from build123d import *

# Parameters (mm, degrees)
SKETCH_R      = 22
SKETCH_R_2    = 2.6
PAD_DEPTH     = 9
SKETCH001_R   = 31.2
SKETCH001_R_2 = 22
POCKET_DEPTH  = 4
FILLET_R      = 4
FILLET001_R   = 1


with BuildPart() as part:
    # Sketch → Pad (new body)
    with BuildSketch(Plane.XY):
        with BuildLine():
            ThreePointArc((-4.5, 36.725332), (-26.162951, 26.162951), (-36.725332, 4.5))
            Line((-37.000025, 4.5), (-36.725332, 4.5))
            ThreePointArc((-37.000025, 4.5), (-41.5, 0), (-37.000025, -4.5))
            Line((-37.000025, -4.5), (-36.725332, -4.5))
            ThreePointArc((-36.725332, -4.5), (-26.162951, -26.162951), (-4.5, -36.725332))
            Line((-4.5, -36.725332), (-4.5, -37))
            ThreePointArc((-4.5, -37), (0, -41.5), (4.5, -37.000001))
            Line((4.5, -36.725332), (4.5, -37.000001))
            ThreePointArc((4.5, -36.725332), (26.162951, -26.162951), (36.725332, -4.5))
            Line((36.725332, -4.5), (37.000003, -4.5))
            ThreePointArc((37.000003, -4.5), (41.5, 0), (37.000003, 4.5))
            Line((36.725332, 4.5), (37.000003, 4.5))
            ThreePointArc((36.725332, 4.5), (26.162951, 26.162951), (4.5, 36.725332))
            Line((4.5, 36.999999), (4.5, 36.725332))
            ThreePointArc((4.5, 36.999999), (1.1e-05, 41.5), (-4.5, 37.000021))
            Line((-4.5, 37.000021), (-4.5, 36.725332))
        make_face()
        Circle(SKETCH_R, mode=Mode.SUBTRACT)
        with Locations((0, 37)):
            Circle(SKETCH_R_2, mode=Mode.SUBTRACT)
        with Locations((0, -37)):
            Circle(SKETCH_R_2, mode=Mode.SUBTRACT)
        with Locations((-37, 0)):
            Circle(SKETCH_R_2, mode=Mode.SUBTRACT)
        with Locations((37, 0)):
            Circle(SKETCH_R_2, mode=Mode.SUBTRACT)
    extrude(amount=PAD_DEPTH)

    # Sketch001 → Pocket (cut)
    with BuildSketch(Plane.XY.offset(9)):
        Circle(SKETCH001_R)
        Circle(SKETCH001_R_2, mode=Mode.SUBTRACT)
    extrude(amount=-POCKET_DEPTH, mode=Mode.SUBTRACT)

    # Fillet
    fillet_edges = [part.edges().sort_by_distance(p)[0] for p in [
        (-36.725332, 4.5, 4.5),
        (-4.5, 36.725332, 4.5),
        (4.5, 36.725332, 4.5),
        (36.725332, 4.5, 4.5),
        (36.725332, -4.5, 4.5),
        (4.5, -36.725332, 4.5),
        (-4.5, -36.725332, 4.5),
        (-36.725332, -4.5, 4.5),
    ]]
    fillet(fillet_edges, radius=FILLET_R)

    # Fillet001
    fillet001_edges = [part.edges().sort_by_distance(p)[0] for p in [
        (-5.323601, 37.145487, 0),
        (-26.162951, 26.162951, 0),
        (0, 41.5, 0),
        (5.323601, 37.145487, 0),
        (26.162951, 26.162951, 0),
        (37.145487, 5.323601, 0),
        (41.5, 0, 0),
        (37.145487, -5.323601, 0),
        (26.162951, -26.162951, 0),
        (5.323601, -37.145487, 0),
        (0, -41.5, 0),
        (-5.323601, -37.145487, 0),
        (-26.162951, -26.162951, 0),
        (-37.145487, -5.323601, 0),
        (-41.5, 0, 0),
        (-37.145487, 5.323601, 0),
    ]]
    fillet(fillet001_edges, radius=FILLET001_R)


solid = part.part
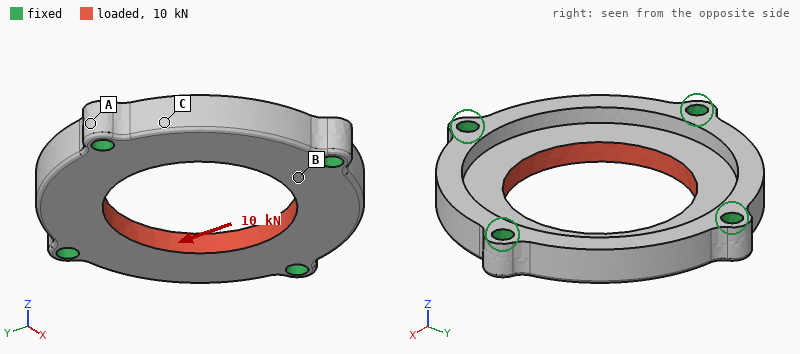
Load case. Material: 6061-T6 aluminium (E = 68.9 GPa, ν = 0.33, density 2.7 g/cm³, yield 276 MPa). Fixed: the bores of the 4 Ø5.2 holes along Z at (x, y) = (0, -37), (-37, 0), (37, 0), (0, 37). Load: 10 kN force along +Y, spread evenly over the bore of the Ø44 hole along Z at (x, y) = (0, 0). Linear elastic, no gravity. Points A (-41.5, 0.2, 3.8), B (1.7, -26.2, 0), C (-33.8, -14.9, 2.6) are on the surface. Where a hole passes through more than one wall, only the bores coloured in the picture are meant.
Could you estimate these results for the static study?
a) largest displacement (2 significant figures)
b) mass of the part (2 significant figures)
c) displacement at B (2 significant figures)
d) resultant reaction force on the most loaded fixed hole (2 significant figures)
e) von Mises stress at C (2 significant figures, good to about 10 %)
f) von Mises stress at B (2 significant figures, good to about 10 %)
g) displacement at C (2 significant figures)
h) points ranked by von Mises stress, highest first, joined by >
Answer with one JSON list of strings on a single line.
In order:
["16 µm", "52 g", "5.8 µm", "2.6 kN", "22 MPa", "36 MPa", "8.7 µm", "B > C > A"]
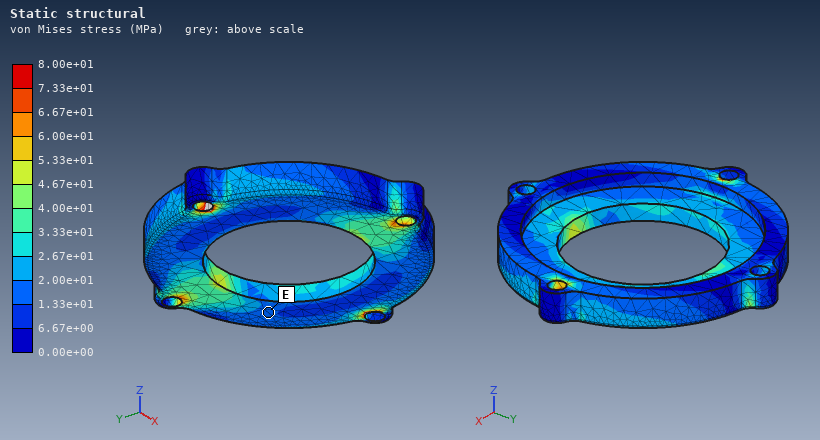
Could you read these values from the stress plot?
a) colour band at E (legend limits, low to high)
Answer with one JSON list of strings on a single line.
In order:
["1.33e+01 to 2.00e+01 MPa"]
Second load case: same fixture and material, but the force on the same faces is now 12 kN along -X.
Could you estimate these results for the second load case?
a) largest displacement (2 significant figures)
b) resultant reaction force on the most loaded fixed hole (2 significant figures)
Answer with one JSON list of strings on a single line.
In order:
["19 µm", "3.2 kN"]
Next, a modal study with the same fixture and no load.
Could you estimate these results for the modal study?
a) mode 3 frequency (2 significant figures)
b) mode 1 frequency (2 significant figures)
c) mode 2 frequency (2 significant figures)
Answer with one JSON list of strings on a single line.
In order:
["14 kHz", "13 kHz", "14 kHz"]
